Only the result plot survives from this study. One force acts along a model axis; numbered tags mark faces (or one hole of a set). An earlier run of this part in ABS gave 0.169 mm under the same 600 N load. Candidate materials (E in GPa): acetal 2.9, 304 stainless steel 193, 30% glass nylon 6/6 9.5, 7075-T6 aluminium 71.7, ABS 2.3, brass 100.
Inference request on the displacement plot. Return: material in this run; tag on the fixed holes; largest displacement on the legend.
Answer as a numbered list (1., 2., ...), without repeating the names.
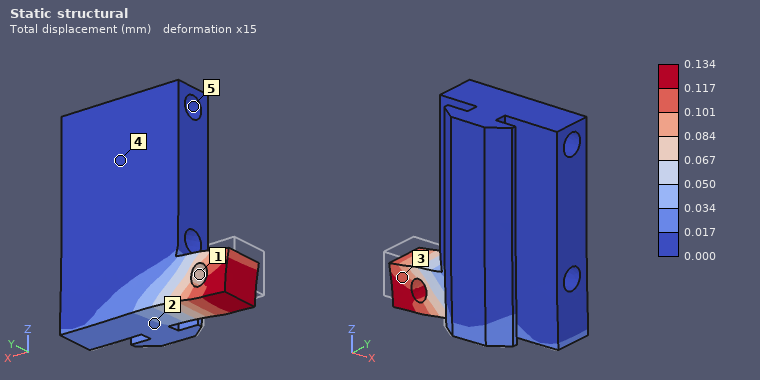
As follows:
1. acetal
2. 5
3. 0.134 mm
